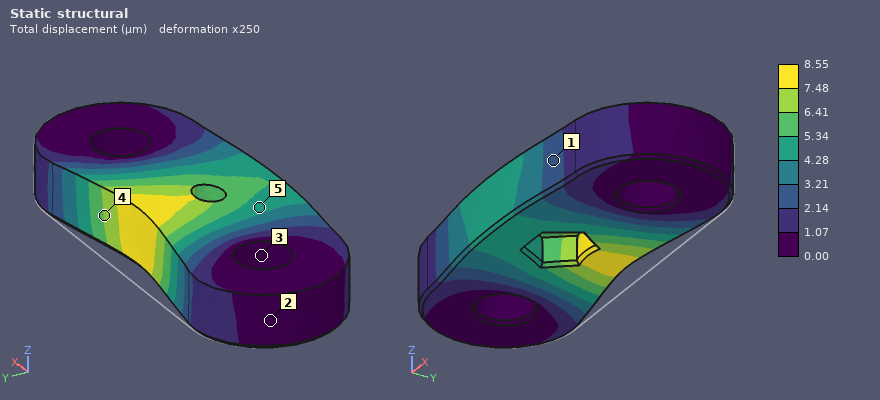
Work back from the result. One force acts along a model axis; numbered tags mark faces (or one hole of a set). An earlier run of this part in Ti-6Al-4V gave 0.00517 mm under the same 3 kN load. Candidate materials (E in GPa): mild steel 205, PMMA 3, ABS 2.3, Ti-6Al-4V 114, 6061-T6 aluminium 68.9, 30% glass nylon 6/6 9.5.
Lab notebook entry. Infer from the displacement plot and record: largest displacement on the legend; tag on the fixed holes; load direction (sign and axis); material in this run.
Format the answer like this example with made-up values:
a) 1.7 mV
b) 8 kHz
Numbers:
a) 8.55 µm
b) 3
c) -Y
d) 6061-T6 aluminium
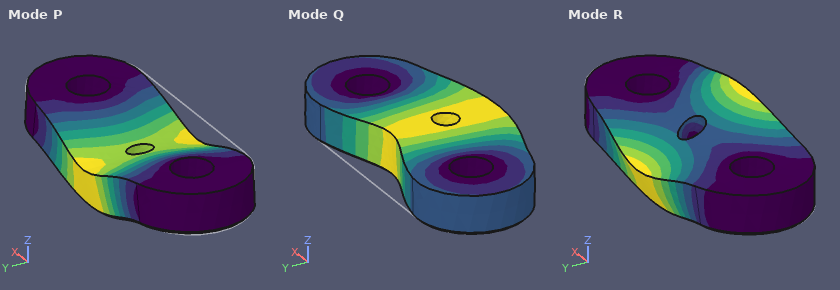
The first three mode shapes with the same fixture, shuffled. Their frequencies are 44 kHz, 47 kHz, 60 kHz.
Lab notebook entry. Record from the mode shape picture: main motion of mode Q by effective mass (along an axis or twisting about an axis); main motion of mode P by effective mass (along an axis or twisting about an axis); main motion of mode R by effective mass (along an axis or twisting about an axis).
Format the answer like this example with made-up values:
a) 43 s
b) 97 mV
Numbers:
a) along Y
b) along Z
c) twisting about X
